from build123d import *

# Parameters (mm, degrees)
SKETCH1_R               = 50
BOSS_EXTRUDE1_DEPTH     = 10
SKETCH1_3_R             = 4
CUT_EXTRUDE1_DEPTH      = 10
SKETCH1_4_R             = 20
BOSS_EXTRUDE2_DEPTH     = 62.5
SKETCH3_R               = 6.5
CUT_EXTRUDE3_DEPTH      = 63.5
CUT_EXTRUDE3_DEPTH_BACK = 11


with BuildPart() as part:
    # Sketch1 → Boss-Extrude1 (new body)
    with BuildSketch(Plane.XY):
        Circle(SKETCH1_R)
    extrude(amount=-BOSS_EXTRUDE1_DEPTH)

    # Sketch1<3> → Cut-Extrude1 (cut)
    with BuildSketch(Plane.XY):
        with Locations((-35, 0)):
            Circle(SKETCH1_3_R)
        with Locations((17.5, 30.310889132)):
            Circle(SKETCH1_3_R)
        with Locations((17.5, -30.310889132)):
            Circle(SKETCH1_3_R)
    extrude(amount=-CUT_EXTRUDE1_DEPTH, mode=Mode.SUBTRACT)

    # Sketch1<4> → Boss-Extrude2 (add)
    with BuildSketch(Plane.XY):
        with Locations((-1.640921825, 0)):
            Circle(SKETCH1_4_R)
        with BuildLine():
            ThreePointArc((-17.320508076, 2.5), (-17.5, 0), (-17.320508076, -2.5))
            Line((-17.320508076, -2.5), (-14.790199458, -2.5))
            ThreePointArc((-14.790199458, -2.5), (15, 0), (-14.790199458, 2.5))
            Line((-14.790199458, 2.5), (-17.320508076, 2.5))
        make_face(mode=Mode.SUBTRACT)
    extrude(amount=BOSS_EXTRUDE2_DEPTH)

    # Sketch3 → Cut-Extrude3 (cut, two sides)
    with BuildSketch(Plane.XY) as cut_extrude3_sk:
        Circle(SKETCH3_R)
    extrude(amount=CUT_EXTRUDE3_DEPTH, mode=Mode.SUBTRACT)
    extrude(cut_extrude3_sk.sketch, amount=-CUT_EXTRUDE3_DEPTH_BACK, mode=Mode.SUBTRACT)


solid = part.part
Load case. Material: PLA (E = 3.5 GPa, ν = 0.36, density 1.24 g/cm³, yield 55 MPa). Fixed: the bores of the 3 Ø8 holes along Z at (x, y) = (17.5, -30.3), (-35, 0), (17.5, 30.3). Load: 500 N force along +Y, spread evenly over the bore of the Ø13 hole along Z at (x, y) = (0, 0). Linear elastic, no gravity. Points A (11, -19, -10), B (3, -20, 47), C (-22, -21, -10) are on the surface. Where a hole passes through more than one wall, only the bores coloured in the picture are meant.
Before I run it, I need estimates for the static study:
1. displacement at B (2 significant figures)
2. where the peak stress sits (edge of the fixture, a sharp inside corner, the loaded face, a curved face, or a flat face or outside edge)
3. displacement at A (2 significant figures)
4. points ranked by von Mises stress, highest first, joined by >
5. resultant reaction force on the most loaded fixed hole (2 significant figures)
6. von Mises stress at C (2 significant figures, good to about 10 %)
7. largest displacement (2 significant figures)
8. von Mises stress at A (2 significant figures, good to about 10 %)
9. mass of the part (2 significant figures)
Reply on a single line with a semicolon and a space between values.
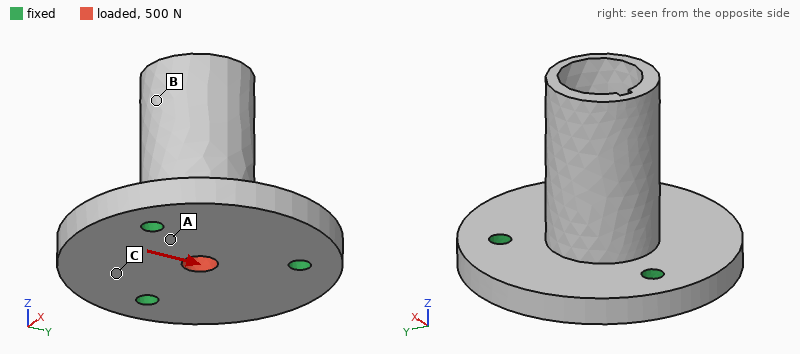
4.0 µm; the loaded face; 3.0 µm; A > C > B; 180 N; 0.33 MPa; 9.7 µm; 0.97 MPa; 140 g
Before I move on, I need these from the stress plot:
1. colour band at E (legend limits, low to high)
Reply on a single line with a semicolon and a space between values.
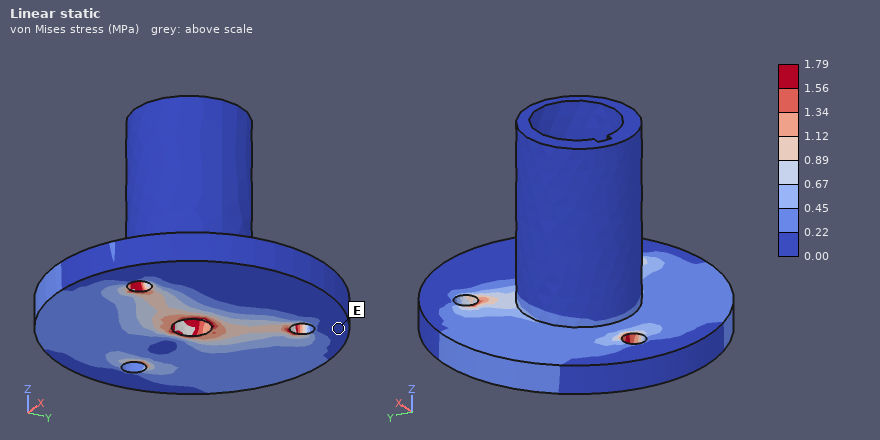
0.00 to 0.22 MPa
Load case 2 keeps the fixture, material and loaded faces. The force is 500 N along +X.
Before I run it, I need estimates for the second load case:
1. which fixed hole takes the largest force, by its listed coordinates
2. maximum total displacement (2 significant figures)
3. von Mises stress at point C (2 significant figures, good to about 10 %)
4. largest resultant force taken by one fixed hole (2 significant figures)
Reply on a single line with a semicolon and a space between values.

(-35, 0); 10 µm; 0.19 MPa; 190 N
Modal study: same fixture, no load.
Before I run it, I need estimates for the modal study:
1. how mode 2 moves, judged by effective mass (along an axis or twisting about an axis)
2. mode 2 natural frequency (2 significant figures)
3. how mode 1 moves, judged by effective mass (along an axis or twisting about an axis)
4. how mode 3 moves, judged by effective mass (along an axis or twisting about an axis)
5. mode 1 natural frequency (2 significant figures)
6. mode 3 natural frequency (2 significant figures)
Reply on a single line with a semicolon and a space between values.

along X; 1400 Hz; along Y; along Z; 1300 Hz; 2600 Hz
